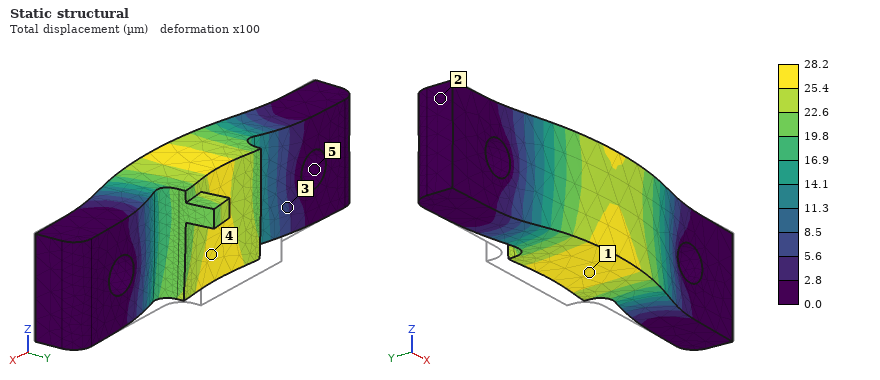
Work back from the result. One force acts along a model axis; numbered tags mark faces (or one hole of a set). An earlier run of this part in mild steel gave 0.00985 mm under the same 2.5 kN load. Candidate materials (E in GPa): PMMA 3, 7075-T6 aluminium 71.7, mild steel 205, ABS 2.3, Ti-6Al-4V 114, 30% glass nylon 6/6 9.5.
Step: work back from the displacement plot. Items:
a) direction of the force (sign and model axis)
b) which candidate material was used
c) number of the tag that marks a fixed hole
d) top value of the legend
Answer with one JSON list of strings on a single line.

["-Y", "7075-T6 aluminium", "5", "28.2 µm"]
